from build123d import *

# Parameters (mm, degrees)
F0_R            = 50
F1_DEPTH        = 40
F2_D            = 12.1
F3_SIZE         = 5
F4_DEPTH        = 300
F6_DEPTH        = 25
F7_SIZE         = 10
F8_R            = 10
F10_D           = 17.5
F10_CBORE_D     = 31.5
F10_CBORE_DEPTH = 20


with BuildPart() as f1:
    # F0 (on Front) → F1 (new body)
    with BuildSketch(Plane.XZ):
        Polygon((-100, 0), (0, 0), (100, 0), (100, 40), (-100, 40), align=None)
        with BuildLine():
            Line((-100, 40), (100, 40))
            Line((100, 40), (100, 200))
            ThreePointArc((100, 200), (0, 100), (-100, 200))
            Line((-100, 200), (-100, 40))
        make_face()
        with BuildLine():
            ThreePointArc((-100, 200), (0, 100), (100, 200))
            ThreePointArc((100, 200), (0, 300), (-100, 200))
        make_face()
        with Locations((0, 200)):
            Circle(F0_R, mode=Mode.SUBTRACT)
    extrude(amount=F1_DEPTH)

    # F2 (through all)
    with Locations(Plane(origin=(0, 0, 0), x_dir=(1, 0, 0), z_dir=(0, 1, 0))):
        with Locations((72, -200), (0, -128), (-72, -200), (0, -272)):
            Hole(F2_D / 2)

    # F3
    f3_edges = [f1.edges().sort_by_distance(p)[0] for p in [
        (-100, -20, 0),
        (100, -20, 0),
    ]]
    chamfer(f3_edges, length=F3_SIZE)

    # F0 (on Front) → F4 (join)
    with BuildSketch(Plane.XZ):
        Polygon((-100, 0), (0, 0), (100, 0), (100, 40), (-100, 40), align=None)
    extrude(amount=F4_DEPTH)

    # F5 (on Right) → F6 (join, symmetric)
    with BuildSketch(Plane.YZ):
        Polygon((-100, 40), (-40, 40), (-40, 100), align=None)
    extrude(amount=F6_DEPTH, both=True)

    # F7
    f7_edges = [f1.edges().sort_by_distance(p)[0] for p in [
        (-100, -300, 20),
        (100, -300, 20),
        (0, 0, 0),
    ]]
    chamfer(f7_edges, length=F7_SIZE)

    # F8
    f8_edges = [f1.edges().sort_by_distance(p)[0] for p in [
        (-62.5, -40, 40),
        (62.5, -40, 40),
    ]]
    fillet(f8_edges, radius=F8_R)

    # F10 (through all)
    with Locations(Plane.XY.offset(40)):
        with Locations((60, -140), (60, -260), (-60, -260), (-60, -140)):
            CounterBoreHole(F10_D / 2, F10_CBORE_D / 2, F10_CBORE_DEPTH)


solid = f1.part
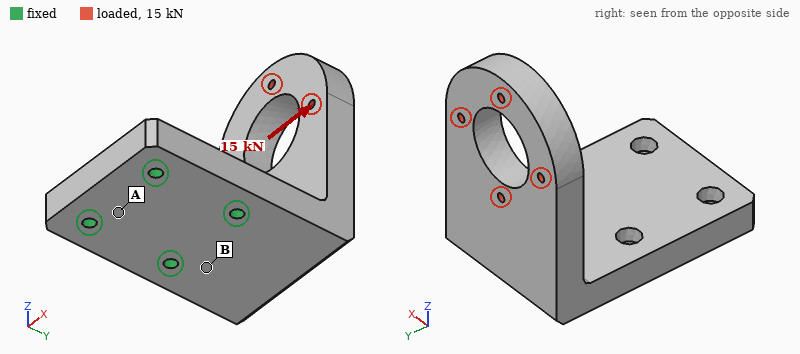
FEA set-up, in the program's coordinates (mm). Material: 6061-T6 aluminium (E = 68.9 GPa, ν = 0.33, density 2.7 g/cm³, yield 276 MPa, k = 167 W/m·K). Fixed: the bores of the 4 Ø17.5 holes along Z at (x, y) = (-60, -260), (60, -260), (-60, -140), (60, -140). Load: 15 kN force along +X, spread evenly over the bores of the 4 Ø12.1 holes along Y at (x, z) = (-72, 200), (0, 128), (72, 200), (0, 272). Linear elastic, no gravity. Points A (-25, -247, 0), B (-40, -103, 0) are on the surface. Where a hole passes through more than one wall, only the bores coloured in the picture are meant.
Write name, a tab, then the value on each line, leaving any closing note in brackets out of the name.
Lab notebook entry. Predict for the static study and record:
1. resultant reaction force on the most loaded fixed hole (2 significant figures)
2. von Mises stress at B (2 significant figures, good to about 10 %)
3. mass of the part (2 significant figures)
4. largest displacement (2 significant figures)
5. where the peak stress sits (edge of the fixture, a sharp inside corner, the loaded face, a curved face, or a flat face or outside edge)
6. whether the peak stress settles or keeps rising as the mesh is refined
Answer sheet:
resultant reaction force on the most loaded fixed hole	29 kN
von Mises stress at B	19 MPa
mass of the part	11 kg
largest displacement	0.51 mm
where the peak stress sits	edge of the fixture
whether the peak stress settles or keeps rising as the mesh is refined	keeps rising
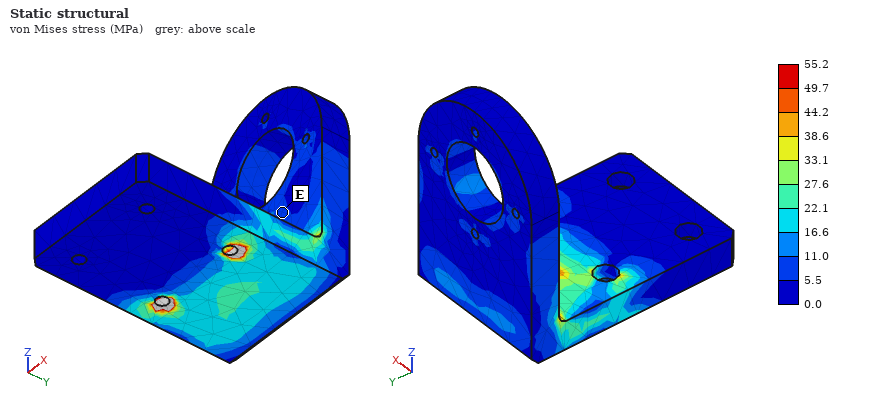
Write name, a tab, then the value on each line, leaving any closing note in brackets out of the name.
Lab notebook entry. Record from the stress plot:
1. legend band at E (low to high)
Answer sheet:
legend band at E	5.5 to 11.0 MPa
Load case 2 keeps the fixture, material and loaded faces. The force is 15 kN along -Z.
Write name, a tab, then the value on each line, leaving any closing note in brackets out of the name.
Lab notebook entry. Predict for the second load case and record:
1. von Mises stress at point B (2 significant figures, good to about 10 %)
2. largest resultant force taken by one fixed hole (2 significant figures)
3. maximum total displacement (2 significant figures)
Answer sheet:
von Mises stress at point B	21 MPa
largest resultant force taken by one fixed hole	15 kN
maximum total displacement	0.60 mm
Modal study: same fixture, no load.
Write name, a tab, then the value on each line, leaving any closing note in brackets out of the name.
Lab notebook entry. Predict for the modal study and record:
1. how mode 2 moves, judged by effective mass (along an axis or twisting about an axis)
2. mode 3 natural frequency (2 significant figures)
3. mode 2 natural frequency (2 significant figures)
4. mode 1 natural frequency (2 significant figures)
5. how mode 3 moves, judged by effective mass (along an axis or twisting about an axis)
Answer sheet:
how mode 2 moves, judged by effective mass	along X
mode 3 natural frequency	980 Hz
mode 2 natural frequency	570 Hz
mode 1 natural frequency	320 Hz
how mode 3 moves, judged by effective mass	along Z
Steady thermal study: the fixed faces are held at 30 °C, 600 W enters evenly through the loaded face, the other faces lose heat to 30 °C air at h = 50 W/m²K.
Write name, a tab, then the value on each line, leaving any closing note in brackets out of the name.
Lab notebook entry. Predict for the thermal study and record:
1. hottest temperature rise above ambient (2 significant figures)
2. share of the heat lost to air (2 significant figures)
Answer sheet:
hottest temperature rise above ambient	82 K
share of the heat lost to air	61 %
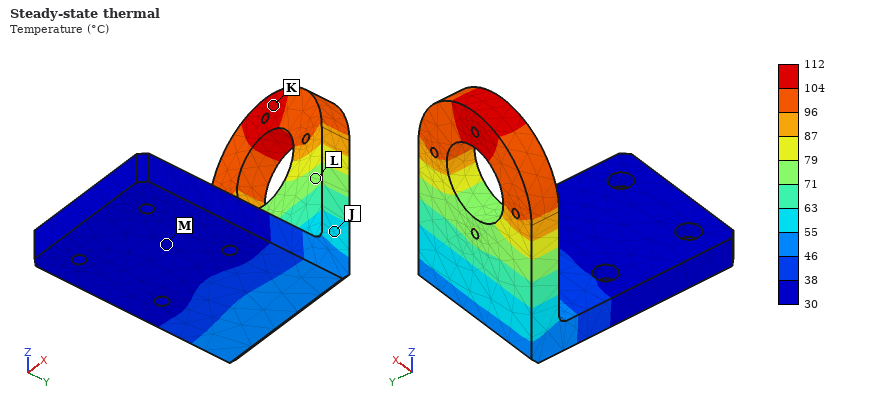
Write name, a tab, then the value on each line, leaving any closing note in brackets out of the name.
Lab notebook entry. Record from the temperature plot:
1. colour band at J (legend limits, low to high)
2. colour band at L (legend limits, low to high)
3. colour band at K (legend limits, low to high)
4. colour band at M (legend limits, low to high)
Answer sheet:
colour band at J	55 to 63 °C
colour band at L	71 to 79 °C
colour band at K	104 to 112 °C
colour band at M	30 to 38 °C
